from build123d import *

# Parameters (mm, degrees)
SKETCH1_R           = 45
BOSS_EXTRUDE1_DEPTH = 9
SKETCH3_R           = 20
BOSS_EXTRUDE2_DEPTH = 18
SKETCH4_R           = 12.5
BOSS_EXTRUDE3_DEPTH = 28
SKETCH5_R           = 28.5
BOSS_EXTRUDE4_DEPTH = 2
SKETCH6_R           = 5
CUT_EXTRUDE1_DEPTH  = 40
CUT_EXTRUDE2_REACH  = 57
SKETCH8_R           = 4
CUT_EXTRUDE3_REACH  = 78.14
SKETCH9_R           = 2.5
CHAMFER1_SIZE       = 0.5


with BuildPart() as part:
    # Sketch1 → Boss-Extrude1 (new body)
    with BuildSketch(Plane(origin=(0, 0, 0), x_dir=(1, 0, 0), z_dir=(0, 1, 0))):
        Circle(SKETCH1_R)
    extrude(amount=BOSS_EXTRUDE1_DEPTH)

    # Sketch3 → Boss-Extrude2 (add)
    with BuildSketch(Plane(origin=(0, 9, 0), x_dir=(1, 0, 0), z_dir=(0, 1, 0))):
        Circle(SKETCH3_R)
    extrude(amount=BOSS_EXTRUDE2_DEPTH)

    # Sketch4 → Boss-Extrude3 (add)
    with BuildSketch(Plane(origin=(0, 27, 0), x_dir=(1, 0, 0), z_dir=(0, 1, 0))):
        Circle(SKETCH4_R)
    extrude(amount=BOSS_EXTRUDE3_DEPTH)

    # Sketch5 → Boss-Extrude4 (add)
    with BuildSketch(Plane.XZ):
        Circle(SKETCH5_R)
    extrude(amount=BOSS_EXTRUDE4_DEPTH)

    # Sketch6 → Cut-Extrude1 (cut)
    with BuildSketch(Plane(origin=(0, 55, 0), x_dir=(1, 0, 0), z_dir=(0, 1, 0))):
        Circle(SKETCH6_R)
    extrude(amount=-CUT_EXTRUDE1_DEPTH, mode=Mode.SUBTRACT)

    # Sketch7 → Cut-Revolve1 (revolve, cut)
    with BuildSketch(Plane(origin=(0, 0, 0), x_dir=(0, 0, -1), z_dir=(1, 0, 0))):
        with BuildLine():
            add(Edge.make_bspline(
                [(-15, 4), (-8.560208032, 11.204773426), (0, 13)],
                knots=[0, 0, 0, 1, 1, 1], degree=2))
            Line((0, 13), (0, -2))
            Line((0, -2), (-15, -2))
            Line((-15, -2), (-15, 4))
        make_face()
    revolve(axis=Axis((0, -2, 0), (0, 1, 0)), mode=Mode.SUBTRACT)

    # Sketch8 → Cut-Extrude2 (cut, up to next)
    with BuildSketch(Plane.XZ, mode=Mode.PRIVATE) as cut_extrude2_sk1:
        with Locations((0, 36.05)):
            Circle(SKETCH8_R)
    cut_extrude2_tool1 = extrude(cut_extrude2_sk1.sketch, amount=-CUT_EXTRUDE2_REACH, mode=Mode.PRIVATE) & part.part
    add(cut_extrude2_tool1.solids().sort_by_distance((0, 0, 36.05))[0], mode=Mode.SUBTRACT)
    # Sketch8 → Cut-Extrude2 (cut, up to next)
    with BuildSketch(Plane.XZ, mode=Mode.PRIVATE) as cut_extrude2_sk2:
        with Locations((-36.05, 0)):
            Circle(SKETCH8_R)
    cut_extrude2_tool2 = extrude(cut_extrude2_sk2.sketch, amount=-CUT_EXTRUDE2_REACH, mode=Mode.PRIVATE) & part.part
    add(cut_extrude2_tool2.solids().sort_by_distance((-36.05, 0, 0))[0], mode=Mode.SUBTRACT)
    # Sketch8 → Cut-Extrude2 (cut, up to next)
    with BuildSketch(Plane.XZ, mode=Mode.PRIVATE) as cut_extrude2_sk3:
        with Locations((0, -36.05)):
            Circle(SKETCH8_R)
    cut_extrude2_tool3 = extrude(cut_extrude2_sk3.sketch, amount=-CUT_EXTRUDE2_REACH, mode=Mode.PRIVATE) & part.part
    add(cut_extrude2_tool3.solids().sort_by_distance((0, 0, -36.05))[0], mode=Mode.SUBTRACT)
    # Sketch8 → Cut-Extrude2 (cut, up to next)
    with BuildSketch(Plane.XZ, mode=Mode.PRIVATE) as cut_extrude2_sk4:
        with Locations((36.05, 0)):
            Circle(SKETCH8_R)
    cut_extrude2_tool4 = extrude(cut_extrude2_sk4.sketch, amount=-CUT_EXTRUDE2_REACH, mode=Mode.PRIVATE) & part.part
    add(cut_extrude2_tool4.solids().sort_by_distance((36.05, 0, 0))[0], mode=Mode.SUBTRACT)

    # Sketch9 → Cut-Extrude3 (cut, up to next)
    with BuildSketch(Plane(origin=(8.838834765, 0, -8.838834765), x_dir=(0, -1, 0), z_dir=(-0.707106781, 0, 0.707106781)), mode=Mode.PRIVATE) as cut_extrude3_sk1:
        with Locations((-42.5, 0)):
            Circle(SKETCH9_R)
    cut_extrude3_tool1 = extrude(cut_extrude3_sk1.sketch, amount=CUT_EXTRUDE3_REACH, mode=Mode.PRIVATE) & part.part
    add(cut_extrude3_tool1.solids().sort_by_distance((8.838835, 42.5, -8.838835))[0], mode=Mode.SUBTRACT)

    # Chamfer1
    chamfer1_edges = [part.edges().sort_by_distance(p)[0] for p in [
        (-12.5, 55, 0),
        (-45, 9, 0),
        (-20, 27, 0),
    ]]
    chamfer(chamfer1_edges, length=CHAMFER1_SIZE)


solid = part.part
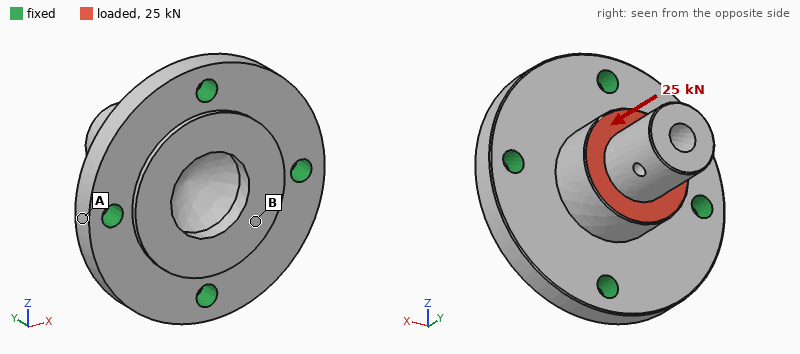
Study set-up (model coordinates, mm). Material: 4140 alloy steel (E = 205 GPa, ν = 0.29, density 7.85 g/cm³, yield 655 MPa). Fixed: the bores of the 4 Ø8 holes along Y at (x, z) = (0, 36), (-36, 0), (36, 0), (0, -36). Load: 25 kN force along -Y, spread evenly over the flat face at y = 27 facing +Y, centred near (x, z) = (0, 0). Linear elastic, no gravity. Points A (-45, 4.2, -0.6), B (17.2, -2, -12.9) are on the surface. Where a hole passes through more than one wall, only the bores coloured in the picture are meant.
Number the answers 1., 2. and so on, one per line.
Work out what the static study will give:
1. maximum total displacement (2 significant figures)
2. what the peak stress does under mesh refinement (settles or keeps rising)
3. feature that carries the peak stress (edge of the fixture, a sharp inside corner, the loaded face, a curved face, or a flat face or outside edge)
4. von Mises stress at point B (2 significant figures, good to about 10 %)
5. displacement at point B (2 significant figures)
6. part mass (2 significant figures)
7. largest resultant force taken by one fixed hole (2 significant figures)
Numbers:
1. 19 µm
2. keeps rising
3. edge of the fixture
4. 57 MPa
5. 14 µm
6. 680 g
7. 6.5 kN
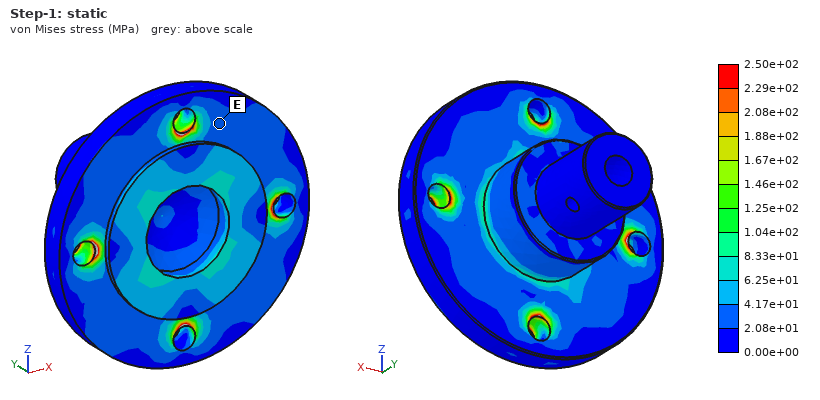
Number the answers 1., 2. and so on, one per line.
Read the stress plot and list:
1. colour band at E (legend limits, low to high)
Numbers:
1. 2.08e+01 to 4.17e+01 MPa
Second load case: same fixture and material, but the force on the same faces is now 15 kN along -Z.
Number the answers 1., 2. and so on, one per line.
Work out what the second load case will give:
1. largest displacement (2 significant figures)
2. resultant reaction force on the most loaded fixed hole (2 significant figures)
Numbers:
1. 33 µm
2. 7.1 kN
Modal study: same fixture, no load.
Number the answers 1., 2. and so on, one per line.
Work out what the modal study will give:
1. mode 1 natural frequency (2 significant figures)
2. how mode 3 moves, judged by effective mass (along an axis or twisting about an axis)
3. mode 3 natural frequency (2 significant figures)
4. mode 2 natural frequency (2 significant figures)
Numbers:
1. 7300 Hz
2. along Y
3. 9900 Hz
4. 7300 Hz
